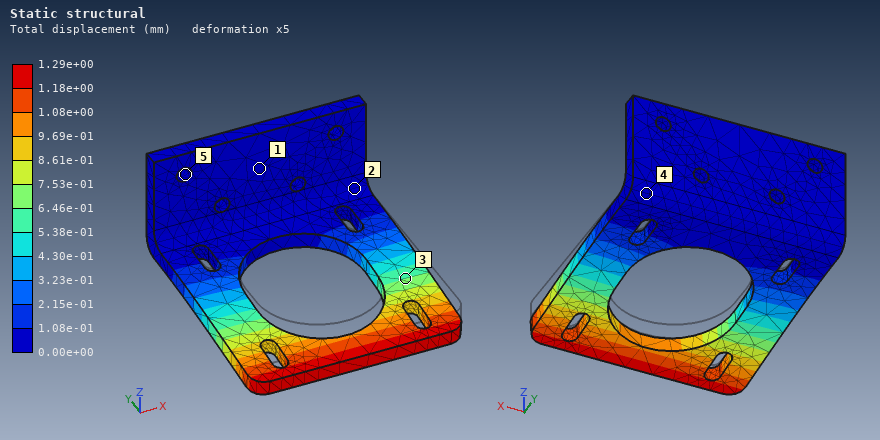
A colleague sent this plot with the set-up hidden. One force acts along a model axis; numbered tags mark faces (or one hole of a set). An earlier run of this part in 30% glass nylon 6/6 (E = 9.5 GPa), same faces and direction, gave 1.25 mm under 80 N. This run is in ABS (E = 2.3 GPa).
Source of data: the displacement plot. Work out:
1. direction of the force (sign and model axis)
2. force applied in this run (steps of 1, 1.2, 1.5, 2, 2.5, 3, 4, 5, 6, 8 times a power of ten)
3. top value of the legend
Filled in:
-Z
20 N
1.29e+00 mm
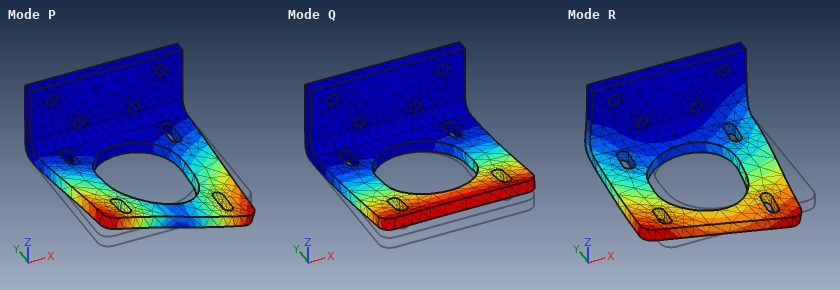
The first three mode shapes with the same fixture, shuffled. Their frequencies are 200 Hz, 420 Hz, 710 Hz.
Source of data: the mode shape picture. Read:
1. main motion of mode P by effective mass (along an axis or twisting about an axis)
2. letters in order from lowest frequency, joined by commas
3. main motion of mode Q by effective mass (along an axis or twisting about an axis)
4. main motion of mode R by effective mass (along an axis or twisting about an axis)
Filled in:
twisting about Y
Q, P, R
along Z
along X
